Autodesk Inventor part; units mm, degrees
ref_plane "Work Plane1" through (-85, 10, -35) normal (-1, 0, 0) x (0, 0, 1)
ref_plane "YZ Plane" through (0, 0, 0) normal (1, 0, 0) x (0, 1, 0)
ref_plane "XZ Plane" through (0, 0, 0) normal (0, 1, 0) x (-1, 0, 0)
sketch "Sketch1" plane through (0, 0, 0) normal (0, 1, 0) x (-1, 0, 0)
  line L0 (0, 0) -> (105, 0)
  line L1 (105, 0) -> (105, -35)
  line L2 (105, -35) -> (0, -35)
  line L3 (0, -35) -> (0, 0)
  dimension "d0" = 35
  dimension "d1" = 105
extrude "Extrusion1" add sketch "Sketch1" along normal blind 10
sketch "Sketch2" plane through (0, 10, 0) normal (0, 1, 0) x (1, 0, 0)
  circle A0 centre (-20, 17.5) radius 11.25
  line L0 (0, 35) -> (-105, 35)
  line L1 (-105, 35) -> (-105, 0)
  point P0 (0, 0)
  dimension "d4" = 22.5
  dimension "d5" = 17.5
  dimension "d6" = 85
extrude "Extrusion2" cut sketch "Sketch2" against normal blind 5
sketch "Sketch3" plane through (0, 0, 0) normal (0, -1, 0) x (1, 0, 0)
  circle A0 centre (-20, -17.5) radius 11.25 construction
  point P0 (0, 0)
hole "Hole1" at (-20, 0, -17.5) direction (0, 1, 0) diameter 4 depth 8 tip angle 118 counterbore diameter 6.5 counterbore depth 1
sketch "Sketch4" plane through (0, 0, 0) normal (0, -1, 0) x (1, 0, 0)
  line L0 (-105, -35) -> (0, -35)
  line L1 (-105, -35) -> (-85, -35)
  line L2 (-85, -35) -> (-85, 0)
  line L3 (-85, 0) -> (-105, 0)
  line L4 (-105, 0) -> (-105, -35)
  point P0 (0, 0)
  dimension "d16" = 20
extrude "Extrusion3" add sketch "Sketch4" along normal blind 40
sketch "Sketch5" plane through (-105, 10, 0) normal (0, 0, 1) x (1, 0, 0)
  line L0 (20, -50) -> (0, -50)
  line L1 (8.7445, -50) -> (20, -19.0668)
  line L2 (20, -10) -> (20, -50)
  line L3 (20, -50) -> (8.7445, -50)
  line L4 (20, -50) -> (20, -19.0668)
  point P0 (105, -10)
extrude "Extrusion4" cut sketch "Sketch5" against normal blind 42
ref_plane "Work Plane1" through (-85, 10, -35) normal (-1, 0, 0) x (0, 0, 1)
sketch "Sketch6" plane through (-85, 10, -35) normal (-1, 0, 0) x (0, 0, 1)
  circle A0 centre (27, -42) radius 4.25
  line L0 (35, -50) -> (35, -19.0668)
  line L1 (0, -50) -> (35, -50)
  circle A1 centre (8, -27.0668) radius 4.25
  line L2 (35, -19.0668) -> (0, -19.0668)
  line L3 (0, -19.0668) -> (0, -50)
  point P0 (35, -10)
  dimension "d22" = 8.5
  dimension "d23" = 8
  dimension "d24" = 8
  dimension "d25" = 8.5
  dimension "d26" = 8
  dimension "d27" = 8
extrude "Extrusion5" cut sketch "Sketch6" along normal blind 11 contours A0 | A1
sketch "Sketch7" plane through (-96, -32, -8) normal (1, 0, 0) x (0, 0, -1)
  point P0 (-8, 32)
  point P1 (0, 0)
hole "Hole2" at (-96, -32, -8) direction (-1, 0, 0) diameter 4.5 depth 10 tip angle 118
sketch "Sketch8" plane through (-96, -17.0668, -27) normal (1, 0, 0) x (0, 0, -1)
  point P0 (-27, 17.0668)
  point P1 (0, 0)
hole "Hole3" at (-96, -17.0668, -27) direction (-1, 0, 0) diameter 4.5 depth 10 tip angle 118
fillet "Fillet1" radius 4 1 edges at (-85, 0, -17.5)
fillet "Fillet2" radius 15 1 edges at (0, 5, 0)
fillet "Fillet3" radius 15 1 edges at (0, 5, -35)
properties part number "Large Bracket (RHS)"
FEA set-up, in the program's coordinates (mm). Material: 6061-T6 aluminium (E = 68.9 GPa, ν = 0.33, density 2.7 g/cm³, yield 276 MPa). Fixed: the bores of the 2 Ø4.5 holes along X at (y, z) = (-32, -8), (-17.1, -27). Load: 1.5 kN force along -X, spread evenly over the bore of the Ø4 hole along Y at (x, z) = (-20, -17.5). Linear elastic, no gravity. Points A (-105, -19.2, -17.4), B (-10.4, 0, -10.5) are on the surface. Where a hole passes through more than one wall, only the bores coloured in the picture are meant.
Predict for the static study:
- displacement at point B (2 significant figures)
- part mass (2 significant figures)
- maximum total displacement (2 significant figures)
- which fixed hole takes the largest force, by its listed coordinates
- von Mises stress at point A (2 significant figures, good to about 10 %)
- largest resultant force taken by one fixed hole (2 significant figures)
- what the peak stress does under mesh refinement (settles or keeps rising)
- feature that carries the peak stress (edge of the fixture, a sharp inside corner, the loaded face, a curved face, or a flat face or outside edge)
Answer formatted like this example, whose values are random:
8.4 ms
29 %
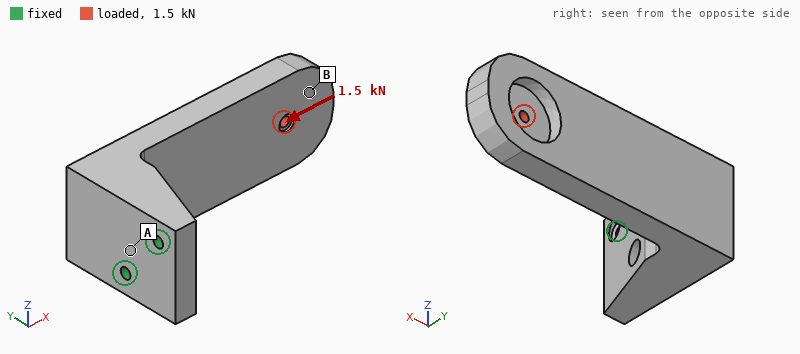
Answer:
85 µm
150 g
91 µm
(-17.1, -27)
14 MPa
1.6 kN
keeps rising
edge of the fixture
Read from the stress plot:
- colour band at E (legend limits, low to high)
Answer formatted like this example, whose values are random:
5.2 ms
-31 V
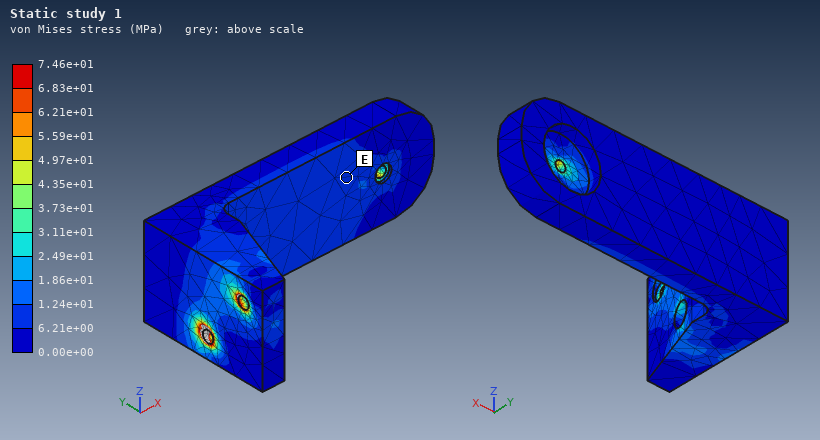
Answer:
6.21e+00 to 1.24e+01 MPa
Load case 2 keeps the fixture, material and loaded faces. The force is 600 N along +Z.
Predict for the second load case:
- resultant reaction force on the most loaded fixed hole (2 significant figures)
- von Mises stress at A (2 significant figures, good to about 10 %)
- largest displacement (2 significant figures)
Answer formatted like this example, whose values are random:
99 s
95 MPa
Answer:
1.5 kN
17 MPa
0.19 mm
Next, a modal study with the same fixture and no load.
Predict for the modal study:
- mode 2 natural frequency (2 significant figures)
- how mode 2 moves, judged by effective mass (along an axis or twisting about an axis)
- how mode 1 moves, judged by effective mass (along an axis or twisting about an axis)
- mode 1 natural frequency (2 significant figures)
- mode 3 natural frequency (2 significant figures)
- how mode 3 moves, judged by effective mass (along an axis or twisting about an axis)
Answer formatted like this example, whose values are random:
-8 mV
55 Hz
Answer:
1700 Hz
along Z
along Y
970 Hz
3800 Hz
along X
